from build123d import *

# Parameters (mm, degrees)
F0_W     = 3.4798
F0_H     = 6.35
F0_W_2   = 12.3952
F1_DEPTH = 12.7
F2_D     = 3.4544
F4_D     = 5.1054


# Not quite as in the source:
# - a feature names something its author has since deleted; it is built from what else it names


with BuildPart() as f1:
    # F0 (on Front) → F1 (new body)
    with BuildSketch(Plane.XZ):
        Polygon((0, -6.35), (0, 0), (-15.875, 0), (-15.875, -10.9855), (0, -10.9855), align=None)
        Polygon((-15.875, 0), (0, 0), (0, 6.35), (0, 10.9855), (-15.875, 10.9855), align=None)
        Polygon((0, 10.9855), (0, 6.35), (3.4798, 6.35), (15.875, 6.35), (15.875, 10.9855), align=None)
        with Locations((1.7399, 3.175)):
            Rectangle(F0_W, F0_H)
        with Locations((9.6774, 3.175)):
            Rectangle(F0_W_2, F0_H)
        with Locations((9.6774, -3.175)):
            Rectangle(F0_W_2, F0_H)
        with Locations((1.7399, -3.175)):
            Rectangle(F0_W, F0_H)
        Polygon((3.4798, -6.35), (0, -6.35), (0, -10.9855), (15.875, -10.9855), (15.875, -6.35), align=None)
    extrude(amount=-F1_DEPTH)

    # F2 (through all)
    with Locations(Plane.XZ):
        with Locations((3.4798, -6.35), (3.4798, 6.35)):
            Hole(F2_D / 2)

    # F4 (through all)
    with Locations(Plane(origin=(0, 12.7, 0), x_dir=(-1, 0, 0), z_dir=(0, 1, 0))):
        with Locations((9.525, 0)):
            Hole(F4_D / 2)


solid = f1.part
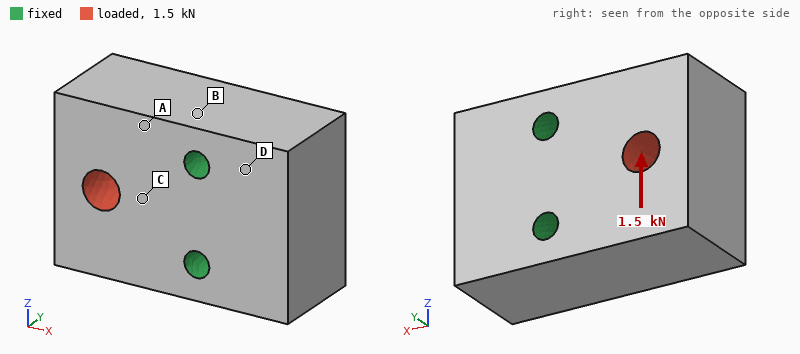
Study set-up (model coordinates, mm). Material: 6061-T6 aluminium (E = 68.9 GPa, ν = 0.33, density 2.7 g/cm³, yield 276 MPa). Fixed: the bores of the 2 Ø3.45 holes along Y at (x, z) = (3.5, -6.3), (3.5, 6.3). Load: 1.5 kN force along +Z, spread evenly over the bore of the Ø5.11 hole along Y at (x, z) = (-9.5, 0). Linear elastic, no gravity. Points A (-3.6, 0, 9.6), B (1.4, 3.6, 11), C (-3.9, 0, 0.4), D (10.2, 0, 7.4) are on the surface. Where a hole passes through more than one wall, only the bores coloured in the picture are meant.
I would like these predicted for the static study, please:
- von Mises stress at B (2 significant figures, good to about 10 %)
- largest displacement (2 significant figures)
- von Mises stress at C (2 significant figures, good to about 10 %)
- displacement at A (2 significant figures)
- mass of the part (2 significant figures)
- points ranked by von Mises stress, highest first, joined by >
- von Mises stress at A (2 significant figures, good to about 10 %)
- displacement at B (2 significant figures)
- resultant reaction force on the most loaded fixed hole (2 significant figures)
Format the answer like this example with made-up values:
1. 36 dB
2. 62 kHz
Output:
1. 13 MPa
2. 7.2 µm
3. 19 MPa
4. 2.8 µm
5. 23 g
6. C > B > A > D
7. 7.5 MPa
8. 1.4 µm
9. 1.5 kN
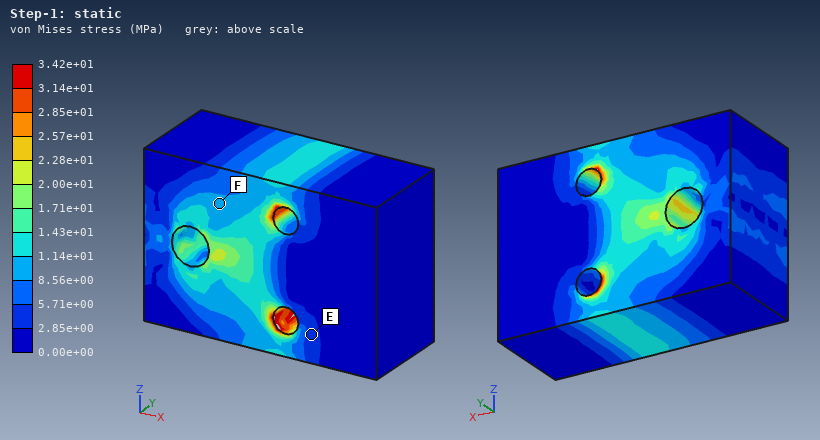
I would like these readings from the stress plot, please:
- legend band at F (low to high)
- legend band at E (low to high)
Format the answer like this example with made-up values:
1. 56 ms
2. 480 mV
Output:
1. 8.56e+00 to 1.14e+01 MPa
2. 2.85e+00 to 5.71e+00 MPa
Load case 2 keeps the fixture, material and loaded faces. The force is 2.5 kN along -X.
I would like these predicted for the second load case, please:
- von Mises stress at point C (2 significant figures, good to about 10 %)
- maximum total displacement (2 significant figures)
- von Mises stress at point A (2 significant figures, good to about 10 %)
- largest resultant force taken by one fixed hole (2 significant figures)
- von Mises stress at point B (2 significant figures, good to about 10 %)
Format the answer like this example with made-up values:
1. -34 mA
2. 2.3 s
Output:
1. 12 MPa
2. 3.9 µm
3. 4.4 MPa
4. 1.3 kN
5. 4.5 MPa
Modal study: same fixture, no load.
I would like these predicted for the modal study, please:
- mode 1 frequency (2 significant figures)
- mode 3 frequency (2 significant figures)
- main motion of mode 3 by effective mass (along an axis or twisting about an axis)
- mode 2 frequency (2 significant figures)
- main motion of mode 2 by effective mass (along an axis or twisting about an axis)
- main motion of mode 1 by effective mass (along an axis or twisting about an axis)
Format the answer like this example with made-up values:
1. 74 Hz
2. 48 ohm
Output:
1. 22 kHz
2. 34 kHz
3. twisting about X
4. 27 kHz
5. along Z
6. along Y
